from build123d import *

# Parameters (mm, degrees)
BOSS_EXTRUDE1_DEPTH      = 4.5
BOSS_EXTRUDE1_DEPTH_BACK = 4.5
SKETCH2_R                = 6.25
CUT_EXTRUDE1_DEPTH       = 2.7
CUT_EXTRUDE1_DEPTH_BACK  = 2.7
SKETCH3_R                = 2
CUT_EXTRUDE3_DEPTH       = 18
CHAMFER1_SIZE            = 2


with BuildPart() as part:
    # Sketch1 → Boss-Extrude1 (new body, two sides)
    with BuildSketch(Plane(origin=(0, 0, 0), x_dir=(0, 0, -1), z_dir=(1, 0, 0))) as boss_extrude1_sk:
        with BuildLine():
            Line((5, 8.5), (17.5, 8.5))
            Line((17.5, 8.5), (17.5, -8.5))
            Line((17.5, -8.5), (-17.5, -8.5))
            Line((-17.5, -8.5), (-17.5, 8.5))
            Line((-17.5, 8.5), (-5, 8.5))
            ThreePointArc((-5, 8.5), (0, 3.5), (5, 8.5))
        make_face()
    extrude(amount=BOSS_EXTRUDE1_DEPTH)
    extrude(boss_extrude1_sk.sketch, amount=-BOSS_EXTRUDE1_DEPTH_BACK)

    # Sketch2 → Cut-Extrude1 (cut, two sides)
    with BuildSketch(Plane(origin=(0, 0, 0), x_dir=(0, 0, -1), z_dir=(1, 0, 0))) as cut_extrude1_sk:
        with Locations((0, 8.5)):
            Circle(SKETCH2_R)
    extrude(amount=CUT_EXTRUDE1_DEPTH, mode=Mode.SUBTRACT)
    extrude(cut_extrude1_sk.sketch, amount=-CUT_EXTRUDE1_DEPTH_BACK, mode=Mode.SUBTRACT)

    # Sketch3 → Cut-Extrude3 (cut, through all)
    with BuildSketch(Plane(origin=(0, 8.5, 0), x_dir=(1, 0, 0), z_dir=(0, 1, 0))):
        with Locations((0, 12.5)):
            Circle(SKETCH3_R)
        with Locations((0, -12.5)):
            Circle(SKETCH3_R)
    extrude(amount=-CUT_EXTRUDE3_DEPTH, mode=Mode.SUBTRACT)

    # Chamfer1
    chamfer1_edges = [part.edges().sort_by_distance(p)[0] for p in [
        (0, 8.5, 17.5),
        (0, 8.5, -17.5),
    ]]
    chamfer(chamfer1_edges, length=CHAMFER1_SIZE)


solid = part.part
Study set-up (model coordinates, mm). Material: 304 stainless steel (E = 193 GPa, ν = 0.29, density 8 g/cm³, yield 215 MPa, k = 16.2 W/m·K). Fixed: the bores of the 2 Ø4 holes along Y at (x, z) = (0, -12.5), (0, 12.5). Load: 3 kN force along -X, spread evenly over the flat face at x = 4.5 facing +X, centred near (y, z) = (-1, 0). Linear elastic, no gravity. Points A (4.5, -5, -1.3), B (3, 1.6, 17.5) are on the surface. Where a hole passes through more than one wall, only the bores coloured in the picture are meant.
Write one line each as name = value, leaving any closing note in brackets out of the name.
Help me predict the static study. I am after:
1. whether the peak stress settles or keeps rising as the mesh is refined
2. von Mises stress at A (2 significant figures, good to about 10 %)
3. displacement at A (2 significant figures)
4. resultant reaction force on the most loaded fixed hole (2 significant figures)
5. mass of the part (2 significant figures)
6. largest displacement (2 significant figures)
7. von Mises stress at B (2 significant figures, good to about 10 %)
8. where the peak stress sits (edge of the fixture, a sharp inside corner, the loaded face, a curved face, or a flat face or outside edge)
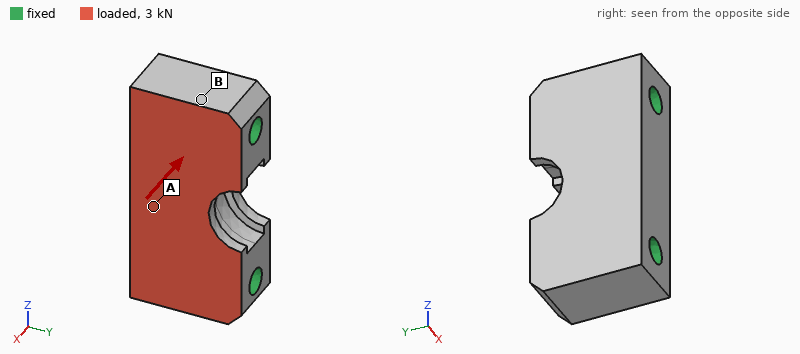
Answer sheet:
whether the peak stress settles or keeps rising as the mesh is refined = keeps rising
von Mises stress at A = 12 MPa
displacement at A = 1.1 µm
resultant reaction force on the most loaded fixed hole = 1.5 kN
mass of the part = 35 g
largest displacement = 1.3 µm
von Mises stress at B = 4.5 MPa
where the peak stress sits = edge of the fixture
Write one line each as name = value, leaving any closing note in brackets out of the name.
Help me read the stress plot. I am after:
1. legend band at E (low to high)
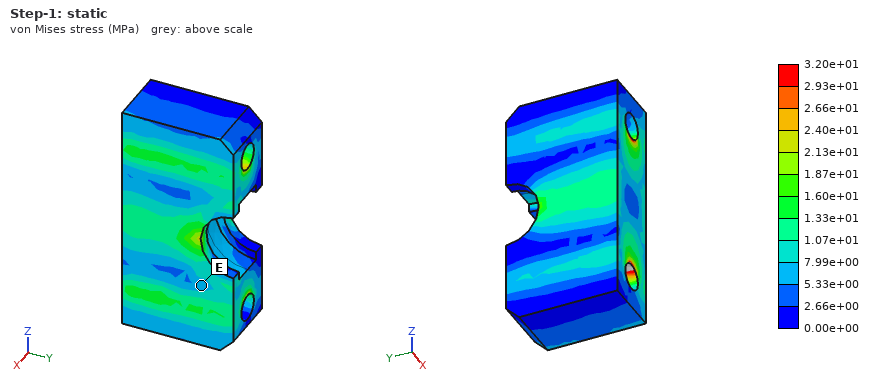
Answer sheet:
legend band at E = 5.33e+00 to 7.99e+00 MPa
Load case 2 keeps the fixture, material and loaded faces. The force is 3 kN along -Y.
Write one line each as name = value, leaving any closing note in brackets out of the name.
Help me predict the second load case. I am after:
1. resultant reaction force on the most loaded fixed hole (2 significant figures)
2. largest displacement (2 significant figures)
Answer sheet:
resultant reaction force on the most loaded fixed hole = 1.5 kN
largest displacement = 1.8 µm
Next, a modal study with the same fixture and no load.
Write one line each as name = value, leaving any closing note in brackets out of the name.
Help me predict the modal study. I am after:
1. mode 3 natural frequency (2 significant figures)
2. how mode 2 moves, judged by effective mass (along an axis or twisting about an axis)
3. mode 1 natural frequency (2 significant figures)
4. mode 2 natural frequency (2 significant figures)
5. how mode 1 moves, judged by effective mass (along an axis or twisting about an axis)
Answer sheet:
mode 3 natural frequency = 70 kHz
how mode 2 moves, judged by effective mass = along Y
mode 1 natural frequency = 47 kHz
mode 2 natural frequency = 63 kHz
how mode 1 moves, judged by effective mass = along X
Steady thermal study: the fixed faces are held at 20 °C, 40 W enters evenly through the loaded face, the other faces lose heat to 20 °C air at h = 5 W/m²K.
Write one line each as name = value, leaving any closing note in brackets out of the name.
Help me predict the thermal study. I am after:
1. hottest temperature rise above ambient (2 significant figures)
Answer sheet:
hottest temperature rise above ambient = 48 K
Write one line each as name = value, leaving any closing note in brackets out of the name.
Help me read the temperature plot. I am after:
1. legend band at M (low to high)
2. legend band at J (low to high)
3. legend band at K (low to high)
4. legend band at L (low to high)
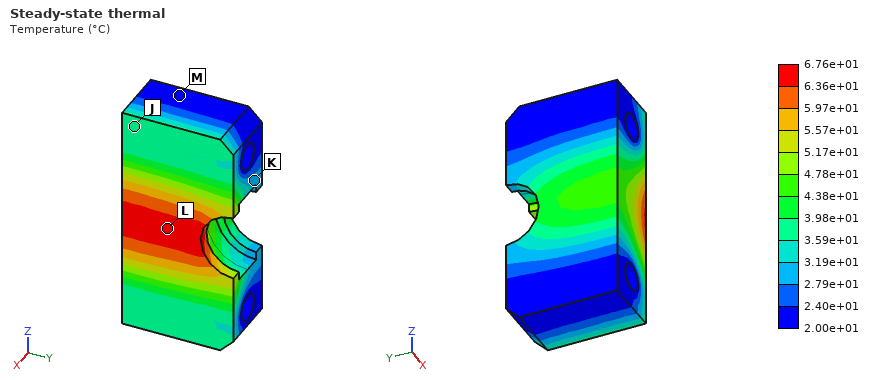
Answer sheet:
legend band at M = 2.00e+01 to 2.40e+01 °C
legend band at J = 3.59e+01 to 3.98e+01 °C
legend band at K = 2.79e+01 to 3.19e+01 °C
legend band at L = 6.36e+01 to 6.76e+01 °C
